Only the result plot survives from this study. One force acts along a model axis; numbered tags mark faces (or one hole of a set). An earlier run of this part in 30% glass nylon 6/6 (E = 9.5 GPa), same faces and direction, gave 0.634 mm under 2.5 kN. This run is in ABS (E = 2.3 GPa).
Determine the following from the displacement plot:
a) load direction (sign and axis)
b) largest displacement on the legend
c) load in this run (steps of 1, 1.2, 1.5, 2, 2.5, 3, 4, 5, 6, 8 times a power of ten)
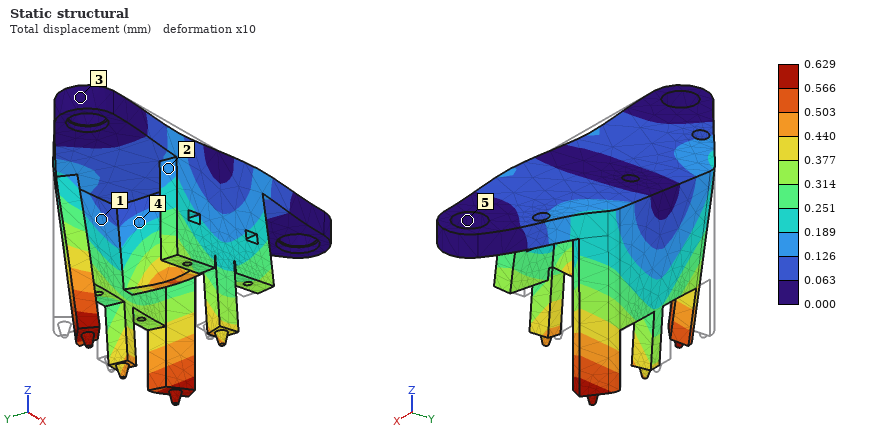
+X
0.629 mm
600 N
